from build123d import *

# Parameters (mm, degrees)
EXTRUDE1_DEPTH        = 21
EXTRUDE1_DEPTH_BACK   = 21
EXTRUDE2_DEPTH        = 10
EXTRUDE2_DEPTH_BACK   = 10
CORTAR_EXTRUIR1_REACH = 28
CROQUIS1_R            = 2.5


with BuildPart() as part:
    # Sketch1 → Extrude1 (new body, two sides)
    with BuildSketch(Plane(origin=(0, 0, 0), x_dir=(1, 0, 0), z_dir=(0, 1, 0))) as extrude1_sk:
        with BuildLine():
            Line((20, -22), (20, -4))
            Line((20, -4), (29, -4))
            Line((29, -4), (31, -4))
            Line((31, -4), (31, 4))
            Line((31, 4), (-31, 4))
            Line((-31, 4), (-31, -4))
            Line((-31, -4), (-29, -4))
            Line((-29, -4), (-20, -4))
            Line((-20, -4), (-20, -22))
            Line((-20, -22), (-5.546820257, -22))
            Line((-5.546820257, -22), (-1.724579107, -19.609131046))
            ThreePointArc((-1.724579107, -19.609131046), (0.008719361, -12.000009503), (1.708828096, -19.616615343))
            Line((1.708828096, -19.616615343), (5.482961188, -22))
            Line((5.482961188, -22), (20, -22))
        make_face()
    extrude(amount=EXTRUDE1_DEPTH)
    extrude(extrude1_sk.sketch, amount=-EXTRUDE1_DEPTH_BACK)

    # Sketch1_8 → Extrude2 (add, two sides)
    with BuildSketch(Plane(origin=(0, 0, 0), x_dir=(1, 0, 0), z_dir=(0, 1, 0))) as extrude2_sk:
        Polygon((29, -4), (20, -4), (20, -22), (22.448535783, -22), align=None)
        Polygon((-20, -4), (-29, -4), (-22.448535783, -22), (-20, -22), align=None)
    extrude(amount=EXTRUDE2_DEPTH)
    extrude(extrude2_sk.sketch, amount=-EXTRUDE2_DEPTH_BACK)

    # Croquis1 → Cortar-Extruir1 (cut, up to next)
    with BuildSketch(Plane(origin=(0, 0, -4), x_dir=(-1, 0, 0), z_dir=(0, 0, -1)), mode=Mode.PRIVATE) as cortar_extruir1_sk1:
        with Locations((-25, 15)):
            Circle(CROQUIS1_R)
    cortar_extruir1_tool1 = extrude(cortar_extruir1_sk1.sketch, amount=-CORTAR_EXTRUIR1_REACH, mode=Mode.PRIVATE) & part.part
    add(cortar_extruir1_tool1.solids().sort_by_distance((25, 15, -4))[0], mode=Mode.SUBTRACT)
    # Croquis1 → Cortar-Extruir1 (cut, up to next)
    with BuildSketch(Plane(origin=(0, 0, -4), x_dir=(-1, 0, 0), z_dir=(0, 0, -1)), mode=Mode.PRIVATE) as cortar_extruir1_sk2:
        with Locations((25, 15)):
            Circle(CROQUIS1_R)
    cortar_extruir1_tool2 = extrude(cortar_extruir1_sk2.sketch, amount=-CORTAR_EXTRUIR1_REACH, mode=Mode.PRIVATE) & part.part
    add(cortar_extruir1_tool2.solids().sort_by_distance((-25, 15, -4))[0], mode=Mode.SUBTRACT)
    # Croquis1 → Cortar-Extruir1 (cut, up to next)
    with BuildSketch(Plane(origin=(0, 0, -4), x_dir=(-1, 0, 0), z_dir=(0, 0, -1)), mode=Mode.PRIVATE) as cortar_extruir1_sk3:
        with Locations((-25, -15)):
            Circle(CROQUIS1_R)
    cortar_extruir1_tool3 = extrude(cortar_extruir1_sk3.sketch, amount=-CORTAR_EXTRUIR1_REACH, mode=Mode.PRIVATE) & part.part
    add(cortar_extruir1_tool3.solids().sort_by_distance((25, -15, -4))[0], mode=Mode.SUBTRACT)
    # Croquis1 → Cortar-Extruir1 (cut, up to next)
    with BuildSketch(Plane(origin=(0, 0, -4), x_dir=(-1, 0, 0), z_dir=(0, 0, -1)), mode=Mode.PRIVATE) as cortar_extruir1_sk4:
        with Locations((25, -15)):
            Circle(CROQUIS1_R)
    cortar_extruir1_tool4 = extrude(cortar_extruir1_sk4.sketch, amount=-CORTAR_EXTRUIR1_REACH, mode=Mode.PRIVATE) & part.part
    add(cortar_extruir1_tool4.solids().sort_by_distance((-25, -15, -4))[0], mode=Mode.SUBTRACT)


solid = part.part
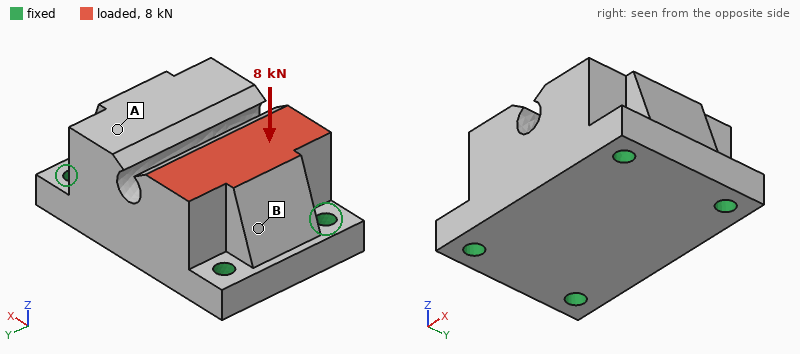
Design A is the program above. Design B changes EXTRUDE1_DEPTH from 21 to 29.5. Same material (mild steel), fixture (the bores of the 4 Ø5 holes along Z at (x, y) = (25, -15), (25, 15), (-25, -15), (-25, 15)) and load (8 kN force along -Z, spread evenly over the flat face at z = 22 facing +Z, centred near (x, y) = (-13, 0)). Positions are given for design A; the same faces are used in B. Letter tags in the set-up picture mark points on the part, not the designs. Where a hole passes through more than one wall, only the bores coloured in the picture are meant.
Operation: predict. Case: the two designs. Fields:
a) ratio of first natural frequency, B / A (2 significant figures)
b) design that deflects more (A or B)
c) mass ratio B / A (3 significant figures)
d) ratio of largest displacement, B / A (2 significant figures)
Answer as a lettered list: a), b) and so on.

a) 0.86
b) B
c) 1.19
d) 1.2
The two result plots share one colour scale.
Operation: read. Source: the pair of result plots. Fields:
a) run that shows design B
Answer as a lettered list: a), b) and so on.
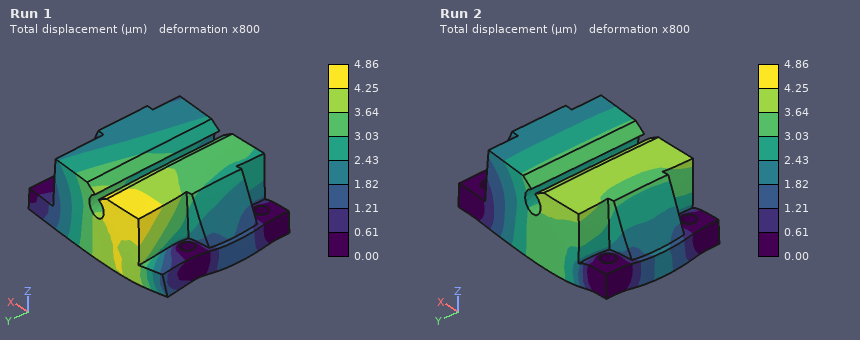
a) Run 1
